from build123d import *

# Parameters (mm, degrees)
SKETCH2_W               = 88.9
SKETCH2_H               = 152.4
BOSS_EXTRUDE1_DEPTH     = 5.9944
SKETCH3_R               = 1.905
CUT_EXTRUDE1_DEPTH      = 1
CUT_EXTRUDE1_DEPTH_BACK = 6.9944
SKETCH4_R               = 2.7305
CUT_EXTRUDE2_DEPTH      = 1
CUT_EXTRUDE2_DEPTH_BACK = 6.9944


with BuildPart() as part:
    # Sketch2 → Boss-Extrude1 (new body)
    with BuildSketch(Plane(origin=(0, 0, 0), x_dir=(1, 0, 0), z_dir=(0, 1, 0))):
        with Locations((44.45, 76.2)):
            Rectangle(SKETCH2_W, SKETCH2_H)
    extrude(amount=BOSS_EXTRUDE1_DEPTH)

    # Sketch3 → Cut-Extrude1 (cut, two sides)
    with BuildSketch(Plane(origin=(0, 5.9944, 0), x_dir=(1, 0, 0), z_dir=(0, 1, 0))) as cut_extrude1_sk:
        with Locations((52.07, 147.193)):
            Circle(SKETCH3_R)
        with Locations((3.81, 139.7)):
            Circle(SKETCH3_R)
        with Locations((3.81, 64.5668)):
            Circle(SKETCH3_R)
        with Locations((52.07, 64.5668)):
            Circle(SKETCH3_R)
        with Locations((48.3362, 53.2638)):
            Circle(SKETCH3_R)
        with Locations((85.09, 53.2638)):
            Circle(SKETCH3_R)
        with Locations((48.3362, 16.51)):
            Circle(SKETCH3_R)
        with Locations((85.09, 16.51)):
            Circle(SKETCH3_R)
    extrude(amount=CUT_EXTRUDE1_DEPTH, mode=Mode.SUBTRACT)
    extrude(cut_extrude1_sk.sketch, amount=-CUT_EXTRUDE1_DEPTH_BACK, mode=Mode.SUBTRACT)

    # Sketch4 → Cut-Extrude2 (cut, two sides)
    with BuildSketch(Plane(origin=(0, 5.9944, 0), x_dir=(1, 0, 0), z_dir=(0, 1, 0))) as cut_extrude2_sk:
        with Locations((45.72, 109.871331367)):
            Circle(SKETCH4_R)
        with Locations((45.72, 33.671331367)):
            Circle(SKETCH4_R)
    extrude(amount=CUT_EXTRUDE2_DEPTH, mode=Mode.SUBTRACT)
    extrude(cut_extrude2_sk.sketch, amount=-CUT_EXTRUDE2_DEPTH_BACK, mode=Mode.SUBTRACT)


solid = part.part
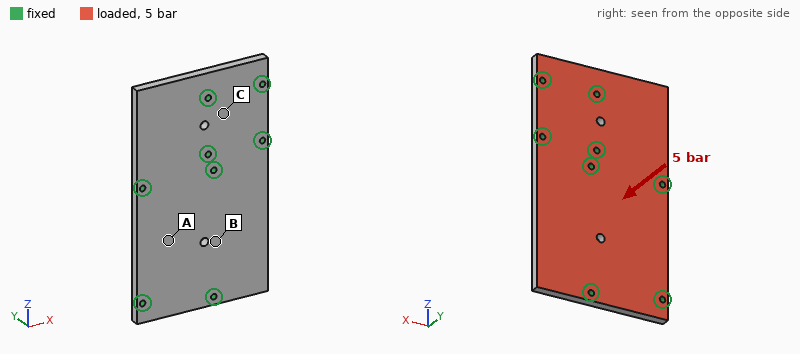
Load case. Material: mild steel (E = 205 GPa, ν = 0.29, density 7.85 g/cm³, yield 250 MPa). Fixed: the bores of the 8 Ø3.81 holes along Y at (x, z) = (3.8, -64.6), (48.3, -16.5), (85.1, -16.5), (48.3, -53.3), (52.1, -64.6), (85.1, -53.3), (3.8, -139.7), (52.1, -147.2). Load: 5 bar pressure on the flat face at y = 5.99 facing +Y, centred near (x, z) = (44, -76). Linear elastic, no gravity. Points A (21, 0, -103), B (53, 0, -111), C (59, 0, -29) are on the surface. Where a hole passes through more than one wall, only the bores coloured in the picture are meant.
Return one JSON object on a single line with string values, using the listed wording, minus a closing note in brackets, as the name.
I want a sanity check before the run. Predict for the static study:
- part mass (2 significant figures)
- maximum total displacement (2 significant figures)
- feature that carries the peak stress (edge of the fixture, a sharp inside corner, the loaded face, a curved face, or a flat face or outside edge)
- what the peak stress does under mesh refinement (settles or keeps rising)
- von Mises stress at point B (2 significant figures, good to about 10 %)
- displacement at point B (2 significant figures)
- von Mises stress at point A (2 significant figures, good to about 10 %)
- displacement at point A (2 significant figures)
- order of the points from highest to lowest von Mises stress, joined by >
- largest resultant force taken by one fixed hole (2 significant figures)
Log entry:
{"part mass": "630 g", "maximum total displacement": "59 µm", "feature that carries the peak stress": "edge of the fixture", "what the peak stress does under mesh refinement": "keeps rising", "von Mises stress at point B": "33 MPa", "displacement at point B": "28 µm", "von Mises stress at point A": "21 MPa", "displacement at point A": "18 µm", "order of the points from highest to lowest von Mises stress, joined by >": "B > A > C", "largest resultant force taken by one fixed hole": "1.4 kN"}
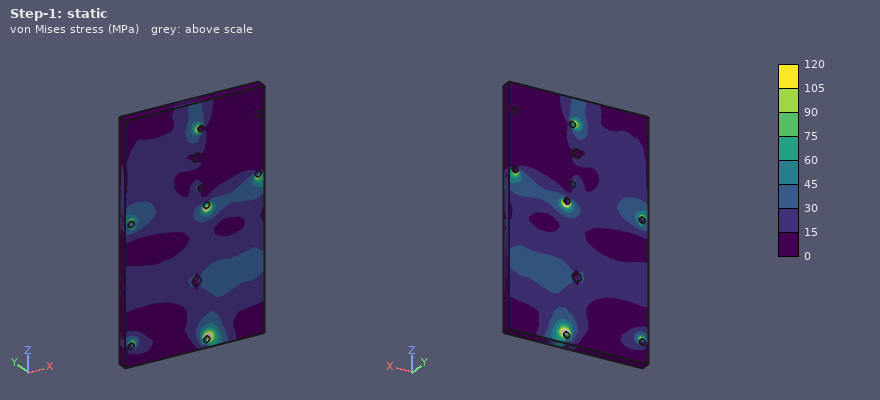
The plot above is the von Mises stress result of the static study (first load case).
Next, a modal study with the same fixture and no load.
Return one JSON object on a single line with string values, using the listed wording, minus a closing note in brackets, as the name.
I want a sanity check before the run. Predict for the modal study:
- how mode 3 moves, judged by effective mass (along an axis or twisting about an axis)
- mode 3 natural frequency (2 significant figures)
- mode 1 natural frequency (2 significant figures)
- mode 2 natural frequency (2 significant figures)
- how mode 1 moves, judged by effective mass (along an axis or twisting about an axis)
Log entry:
{"how mode 3 moves, judged by effective mass": "along Y", "mode 3 natural frequency": "4400 Hz", "mode 1 natural frequency": "2800 Hz", "mode 2 natural frequency": "3000 Hz", "how mode 1 moves, judged by effective mass": "along Y"}
